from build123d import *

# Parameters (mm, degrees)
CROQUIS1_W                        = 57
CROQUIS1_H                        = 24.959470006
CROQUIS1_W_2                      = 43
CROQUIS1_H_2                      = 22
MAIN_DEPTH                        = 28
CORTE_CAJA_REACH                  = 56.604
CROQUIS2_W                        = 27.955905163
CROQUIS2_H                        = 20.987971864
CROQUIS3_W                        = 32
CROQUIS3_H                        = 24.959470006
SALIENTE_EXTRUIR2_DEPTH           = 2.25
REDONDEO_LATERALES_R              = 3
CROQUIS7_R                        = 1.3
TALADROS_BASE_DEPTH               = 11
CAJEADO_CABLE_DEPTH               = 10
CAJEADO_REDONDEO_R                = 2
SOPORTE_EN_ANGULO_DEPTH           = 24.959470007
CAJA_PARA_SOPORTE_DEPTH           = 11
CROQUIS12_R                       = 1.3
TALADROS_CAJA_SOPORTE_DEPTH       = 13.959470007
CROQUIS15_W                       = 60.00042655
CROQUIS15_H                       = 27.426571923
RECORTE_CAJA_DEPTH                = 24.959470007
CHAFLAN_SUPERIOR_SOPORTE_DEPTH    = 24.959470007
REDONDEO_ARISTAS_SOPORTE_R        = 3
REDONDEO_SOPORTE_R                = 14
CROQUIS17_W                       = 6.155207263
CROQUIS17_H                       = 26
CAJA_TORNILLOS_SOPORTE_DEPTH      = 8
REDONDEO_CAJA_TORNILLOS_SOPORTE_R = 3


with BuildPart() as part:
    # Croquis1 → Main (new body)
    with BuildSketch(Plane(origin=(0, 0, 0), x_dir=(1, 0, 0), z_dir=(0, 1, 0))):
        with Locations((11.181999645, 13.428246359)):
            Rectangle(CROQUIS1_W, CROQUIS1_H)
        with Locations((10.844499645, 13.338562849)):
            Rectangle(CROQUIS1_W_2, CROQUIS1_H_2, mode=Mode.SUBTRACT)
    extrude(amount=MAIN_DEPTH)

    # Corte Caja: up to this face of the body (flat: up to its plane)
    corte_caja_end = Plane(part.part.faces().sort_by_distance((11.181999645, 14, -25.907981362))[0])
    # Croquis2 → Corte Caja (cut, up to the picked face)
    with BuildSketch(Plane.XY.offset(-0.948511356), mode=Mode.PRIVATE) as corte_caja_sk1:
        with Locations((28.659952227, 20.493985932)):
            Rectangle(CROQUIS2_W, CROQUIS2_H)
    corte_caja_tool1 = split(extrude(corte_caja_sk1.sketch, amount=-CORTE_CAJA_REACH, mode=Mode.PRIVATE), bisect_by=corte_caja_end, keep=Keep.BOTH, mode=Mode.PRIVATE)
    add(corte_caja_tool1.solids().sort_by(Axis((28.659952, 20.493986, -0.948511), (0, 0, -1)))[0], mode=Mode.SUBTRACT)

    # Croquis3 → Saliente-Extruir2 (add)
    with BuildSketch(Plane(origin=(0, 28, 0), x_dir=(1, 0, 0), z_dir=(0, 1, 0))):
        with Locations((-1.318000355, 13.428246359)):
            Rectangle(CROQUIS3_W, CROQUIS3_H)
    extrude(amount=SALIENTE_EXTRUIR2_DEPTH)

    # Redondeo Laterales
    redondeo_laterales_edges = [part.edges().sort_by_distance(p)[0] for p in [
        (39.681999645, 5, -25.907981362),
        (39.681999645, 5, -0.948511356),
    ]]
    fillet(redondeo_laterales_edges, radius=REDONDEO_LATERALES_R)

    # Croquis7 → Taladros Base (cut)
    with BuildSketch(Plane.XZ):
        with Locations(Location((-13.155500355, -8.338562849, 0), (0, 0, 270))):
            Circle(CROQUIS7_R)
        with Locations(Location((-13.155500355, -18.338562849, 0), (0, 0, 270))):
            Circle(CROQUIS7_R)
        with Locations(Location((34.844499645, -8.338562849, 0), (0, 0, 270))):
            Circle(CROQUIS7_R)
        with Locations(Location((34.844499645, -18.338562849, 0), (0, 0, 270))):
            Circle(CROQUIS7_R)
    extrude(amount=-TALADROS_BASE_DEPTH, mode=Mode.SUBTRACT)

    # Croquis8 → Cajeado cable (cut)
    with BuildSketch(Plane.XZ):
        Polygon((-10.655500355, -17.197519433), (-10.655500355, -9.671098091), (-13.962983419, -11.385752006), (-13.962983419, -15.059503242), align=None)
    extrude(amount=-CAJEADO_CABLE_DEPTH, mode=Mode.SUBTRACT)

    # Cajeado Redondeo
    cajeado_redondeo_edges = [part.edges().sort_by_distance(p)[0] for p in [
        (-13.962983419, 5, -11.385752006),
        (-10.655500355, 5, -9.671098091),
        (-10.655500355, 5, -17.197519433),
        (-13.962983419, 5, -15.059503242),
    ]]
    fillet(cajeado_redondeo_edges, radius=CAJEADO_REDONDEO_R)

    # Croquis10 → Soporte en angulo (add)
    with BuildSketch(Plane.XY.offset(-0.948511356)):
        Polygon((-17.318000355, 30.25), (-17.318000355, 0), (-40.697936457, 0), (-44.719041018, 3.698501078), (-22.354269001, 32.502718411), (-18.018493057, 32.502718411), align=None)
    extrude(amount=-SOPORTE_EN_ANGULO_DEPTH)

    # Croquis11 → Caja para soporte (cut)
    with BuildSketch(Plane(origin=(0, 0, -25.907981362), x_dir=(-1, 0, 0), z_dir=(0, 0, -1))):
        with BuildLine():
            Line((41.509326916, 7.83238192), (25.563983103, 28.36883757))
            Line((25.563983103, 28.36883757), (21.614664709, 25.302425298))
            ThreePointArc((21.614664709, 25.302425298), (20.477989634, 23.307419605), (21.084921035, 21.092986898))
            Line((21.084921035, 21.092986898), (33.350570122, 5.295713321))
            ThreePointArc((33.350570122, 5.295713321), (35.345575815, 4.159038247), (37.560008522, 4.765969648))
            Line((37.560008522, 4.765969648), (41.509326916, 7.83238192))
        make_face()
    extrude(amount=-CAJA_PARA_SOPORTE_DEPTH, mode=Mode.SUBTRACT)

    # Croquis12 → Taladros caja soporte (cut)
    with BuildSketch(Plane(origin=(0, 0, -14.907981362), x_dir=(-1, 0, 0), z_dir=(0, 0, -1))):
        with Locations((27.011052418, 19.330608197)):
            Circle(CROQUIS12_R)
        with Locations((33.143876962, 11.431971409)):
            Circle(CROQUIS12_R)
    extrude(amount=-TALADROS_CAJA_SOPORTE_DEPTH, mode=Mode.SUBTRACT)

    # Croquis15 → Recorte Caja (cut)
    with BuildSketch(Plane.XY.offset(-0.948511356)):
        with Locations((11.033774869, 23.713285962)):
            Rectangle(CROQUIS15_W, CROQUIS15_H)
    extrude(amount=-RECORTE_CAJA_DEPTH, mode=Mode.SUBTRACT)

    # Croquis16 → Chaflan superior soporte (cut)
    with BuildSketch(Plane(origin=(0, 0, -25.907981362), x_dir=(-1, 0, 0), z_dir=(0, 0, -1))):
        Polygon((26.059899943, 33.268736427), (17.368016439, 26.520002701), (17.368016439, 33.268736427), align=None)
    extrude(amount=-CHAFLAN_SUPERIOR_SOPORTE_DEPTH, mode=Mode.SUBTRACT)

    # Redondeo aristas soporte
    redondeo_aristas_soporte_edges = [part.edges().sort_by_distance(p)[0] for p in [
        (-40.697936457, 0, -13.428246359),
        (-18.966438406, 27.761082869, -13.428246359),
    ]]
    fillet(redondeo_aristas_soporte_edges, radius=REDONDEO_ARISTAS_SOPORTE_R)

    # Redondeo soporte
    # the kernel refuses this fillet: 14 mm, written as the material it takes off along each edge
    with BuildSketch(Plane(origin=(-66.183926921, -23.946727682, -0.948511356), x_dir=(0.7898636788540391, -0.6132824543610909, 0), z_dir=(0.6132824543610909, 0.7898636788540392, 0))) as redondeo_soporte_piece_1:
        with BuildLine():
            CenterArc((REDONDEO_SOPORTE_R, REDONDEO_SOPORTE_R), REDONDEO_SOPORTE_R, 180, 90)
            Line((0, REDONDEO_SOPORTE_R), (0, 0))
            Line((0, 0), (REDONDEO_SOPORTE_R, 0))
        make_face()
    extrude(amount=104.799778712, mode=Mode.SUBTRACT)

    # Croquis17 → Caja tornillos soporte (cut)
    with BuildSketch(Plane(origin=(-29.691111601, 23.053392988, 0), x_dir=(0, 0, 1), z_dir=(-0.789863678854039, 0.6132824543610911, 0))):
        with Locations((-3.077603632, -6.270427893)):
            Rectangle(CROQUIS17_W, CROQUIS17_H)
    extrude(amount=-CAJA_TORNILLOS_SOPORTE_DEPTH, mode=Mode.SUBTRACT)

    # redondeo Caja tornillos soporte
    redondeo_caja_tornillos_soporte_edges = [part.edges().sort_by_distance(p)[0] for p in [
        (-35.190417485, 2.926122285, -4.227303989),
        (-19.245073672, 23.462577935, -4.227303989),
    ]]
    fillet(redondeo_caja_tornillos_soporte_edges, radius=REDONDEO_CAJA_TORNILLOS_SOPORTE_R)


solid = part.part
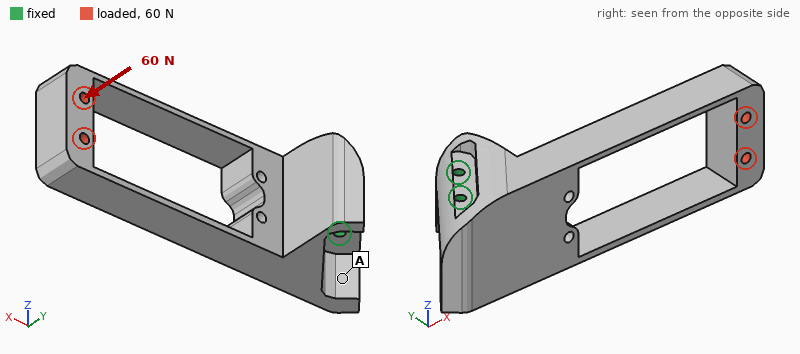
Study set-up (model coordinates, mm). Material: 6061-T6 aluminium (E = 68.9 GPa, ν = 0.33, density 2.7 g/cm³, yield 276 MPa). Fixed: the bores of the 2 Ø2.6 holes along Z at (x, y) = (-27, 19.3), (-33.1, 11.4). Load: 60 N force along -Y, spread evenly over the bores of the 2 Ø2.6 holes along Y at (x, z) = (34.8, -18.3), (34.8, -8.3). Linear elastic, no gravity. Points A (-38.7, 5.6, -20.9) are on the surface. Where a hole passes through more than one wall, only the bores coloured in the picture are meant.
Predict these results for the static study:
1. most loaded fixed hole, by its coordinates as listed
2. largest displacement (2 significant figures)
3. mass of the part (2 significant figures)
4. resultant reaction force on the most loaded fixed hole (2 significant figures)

(-27, 19.3)
0.19 mm
35 g
360 N
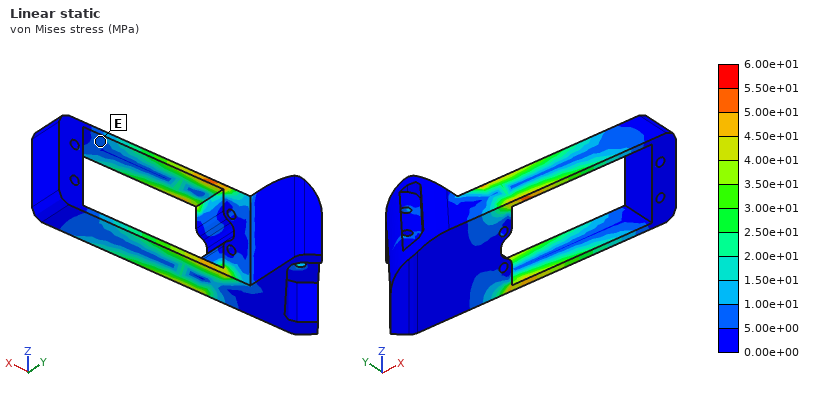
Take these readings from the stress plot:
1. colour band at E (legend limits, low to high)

5.00e+00 to 1.00e+01 MPa
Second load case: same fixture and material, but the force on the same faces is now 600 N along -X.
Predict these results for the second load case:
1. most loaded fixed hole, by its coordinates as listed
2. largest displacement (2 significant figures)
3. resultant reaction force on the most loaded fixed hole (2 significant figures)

(-33.1, 11.4)
29 µm
770 N
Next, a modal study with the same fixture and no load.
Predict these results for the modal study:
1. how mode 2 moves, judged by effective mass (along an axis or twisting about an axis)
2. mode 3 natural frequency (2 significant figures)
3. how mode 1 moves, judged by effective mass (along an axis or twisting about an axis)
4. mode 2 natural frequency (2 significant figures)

along Y
3100 Hz
along Z
1300 Hz
